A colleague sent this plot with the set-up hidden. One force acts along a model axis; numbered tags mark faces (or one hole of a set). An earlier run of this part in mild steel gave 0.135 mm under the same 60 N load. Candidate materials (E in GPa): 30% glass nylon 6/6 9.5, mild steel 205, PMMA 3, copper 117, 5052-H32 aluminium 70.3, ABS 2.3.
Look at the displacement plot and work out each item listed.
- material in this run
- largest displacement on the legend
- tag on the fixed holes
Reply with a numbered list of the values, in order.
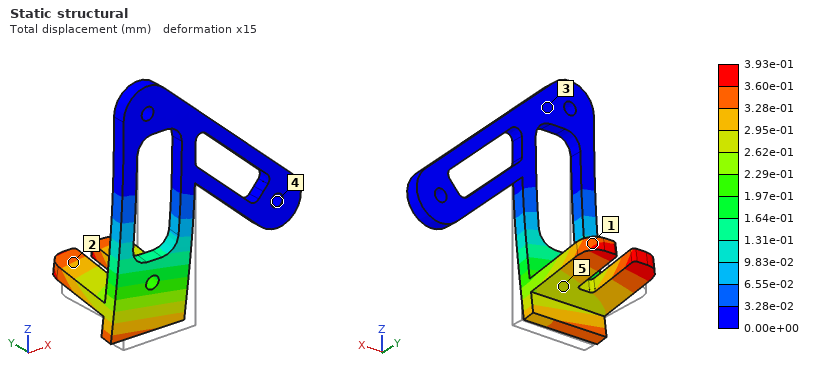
1. 5052-H32 aluminium
2. 3.93e-01 mm
3. 4
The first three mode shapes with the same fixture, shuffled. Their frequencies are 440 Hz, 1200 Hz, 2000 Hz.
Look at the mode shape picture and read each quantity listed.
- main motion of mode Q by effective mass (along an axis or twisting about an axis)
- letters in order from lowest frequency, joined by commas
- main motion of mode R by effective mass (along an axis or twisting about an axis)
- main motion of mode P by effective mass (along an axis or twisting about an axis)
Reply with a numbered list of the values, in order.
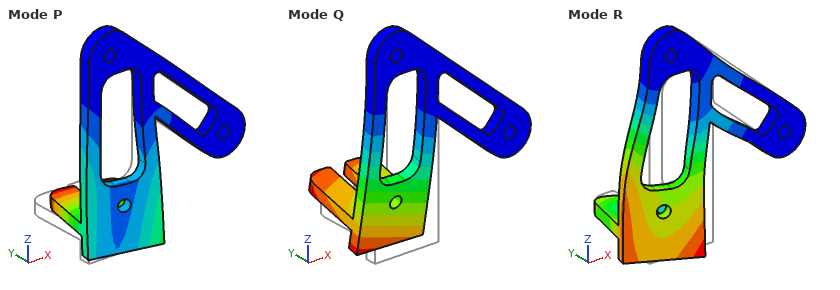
1. along Y
2. Q, P, R
3. along X
4. along X
